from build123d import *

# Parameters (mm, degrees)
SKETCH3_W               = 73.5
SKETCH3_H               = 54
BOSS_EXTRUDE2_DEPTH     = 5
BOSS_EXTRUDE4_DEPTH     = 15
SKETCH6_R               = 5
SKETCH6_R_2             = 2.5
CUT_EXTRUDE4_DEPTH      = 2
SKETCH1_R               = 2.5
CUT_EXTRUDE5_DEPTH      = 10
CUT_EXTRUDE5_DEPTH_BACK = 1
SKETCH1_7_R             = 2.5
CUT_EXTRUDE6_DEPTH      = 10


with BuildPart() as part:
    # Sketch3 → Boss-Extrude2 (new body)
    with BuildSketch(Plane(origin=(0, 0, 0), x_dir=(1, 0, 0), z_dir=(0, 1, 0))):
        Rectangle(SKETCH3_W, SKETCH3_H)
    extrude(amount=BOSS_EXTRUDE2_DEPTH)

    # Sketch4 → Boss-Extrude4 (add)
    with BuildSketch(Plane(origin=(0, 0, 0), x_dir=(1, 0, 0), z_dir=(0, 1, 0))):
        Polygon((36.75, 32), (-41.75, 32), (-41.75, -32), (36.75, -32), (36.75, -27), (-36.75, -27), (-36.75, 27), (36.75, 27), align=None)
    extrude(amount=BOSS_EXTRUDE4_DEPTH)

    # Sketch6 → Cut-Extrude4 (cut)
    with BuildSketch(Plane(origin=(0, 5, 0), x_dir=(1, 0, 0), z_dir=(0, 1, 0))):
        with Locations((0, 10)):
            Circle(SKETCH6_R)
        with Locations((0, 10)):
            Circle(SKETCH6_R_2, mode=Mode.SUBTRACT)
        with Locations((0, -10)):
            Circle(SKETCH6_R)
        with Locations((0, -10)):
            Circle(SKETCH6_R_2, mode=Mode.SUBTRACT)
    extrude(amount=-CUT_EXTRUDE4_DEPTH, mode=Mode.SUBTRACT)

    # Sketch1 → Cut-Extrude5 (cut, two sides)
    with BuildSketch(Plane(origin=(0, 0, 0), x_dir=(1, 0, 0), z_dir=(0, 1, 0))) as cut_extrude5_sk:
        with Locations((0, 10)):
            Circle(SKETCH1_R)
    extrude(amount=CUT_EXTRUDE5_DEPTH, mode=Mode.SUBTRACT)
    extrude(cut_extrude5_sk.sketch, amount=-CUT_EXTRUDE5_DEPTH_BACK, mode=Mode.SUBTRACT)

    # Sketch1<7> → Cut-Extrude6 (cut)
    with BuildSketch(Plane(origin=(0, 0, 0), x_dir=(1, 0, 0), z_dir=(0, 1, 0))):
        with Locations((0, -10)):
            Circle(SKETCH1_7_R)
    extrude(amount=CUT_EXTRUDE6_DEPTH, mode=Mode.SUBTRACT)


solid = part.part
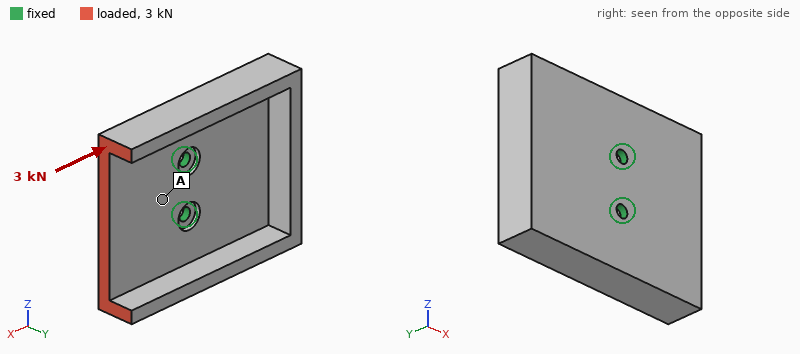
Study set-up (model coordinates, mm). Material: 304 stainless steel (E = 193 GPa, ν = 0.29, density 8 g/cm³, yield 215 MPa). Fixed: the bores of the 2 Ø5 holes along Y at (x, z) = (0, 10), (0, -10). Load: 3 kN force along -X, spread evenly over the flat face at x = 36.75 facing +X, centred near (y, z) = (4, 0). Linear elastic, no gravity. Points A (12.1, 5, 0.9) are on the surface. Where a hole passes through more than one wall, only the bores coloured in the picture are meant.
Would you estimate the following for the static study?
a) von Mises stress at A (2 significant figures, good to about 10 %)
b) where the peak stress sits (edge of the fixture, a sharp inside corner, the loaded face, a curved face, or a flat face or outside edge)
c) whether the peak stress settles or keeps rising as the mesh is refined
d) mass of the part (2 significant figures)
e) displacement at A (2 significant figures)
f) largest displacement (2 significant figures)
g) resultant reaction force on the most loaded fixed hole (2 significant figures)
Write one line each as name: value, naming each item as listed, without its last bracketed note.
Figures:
von Mises stress at A: 15 MPa
where the peak stress sits: edge of the fixture
whether the peak stress settles or keeps rising as the mesh is refined: keeps rising
mass of the part: 280 g
displacement at A: 8.5 µm
largest displacement: 37 µm
resultant reaction force on the most loaded fixed hole: 1.5 kN
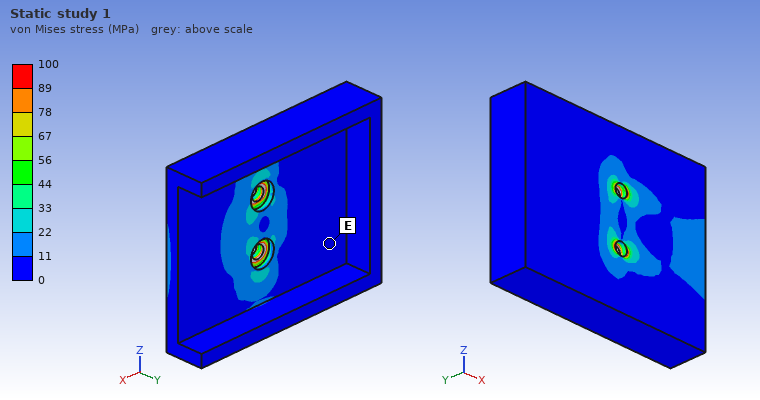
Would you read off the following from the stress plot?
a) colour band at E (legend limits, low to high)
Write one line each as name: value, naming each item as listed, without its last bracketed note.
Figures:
colour band at E: 0 to 11 MPa
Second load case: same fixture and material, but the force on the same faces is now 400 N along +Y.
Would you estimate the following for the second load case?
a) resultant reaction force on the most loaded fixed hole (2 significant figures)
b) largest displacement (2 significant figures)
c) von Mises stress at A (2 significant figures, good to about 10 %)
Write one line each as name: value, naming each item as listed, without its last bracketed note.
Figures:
resultant reaction force on the most loaded fixed hole: 280 N
largest displacement: 68 µm
von Mises stress at A: 25 MPa
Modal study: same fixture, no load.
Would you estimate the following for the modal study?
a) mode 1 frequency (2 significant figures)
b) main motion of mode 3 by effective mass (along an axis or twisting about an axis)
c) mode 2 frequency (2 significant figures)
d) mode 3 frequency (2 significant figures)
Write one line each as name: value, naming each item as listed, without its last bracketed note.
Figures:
mode 1 frequency: 1200 Hz
main motion of mode 3 by effective mass: twisting about X
mode 2 frequency: 2400 Hz
mode 3 frequency: 2900 Hz
